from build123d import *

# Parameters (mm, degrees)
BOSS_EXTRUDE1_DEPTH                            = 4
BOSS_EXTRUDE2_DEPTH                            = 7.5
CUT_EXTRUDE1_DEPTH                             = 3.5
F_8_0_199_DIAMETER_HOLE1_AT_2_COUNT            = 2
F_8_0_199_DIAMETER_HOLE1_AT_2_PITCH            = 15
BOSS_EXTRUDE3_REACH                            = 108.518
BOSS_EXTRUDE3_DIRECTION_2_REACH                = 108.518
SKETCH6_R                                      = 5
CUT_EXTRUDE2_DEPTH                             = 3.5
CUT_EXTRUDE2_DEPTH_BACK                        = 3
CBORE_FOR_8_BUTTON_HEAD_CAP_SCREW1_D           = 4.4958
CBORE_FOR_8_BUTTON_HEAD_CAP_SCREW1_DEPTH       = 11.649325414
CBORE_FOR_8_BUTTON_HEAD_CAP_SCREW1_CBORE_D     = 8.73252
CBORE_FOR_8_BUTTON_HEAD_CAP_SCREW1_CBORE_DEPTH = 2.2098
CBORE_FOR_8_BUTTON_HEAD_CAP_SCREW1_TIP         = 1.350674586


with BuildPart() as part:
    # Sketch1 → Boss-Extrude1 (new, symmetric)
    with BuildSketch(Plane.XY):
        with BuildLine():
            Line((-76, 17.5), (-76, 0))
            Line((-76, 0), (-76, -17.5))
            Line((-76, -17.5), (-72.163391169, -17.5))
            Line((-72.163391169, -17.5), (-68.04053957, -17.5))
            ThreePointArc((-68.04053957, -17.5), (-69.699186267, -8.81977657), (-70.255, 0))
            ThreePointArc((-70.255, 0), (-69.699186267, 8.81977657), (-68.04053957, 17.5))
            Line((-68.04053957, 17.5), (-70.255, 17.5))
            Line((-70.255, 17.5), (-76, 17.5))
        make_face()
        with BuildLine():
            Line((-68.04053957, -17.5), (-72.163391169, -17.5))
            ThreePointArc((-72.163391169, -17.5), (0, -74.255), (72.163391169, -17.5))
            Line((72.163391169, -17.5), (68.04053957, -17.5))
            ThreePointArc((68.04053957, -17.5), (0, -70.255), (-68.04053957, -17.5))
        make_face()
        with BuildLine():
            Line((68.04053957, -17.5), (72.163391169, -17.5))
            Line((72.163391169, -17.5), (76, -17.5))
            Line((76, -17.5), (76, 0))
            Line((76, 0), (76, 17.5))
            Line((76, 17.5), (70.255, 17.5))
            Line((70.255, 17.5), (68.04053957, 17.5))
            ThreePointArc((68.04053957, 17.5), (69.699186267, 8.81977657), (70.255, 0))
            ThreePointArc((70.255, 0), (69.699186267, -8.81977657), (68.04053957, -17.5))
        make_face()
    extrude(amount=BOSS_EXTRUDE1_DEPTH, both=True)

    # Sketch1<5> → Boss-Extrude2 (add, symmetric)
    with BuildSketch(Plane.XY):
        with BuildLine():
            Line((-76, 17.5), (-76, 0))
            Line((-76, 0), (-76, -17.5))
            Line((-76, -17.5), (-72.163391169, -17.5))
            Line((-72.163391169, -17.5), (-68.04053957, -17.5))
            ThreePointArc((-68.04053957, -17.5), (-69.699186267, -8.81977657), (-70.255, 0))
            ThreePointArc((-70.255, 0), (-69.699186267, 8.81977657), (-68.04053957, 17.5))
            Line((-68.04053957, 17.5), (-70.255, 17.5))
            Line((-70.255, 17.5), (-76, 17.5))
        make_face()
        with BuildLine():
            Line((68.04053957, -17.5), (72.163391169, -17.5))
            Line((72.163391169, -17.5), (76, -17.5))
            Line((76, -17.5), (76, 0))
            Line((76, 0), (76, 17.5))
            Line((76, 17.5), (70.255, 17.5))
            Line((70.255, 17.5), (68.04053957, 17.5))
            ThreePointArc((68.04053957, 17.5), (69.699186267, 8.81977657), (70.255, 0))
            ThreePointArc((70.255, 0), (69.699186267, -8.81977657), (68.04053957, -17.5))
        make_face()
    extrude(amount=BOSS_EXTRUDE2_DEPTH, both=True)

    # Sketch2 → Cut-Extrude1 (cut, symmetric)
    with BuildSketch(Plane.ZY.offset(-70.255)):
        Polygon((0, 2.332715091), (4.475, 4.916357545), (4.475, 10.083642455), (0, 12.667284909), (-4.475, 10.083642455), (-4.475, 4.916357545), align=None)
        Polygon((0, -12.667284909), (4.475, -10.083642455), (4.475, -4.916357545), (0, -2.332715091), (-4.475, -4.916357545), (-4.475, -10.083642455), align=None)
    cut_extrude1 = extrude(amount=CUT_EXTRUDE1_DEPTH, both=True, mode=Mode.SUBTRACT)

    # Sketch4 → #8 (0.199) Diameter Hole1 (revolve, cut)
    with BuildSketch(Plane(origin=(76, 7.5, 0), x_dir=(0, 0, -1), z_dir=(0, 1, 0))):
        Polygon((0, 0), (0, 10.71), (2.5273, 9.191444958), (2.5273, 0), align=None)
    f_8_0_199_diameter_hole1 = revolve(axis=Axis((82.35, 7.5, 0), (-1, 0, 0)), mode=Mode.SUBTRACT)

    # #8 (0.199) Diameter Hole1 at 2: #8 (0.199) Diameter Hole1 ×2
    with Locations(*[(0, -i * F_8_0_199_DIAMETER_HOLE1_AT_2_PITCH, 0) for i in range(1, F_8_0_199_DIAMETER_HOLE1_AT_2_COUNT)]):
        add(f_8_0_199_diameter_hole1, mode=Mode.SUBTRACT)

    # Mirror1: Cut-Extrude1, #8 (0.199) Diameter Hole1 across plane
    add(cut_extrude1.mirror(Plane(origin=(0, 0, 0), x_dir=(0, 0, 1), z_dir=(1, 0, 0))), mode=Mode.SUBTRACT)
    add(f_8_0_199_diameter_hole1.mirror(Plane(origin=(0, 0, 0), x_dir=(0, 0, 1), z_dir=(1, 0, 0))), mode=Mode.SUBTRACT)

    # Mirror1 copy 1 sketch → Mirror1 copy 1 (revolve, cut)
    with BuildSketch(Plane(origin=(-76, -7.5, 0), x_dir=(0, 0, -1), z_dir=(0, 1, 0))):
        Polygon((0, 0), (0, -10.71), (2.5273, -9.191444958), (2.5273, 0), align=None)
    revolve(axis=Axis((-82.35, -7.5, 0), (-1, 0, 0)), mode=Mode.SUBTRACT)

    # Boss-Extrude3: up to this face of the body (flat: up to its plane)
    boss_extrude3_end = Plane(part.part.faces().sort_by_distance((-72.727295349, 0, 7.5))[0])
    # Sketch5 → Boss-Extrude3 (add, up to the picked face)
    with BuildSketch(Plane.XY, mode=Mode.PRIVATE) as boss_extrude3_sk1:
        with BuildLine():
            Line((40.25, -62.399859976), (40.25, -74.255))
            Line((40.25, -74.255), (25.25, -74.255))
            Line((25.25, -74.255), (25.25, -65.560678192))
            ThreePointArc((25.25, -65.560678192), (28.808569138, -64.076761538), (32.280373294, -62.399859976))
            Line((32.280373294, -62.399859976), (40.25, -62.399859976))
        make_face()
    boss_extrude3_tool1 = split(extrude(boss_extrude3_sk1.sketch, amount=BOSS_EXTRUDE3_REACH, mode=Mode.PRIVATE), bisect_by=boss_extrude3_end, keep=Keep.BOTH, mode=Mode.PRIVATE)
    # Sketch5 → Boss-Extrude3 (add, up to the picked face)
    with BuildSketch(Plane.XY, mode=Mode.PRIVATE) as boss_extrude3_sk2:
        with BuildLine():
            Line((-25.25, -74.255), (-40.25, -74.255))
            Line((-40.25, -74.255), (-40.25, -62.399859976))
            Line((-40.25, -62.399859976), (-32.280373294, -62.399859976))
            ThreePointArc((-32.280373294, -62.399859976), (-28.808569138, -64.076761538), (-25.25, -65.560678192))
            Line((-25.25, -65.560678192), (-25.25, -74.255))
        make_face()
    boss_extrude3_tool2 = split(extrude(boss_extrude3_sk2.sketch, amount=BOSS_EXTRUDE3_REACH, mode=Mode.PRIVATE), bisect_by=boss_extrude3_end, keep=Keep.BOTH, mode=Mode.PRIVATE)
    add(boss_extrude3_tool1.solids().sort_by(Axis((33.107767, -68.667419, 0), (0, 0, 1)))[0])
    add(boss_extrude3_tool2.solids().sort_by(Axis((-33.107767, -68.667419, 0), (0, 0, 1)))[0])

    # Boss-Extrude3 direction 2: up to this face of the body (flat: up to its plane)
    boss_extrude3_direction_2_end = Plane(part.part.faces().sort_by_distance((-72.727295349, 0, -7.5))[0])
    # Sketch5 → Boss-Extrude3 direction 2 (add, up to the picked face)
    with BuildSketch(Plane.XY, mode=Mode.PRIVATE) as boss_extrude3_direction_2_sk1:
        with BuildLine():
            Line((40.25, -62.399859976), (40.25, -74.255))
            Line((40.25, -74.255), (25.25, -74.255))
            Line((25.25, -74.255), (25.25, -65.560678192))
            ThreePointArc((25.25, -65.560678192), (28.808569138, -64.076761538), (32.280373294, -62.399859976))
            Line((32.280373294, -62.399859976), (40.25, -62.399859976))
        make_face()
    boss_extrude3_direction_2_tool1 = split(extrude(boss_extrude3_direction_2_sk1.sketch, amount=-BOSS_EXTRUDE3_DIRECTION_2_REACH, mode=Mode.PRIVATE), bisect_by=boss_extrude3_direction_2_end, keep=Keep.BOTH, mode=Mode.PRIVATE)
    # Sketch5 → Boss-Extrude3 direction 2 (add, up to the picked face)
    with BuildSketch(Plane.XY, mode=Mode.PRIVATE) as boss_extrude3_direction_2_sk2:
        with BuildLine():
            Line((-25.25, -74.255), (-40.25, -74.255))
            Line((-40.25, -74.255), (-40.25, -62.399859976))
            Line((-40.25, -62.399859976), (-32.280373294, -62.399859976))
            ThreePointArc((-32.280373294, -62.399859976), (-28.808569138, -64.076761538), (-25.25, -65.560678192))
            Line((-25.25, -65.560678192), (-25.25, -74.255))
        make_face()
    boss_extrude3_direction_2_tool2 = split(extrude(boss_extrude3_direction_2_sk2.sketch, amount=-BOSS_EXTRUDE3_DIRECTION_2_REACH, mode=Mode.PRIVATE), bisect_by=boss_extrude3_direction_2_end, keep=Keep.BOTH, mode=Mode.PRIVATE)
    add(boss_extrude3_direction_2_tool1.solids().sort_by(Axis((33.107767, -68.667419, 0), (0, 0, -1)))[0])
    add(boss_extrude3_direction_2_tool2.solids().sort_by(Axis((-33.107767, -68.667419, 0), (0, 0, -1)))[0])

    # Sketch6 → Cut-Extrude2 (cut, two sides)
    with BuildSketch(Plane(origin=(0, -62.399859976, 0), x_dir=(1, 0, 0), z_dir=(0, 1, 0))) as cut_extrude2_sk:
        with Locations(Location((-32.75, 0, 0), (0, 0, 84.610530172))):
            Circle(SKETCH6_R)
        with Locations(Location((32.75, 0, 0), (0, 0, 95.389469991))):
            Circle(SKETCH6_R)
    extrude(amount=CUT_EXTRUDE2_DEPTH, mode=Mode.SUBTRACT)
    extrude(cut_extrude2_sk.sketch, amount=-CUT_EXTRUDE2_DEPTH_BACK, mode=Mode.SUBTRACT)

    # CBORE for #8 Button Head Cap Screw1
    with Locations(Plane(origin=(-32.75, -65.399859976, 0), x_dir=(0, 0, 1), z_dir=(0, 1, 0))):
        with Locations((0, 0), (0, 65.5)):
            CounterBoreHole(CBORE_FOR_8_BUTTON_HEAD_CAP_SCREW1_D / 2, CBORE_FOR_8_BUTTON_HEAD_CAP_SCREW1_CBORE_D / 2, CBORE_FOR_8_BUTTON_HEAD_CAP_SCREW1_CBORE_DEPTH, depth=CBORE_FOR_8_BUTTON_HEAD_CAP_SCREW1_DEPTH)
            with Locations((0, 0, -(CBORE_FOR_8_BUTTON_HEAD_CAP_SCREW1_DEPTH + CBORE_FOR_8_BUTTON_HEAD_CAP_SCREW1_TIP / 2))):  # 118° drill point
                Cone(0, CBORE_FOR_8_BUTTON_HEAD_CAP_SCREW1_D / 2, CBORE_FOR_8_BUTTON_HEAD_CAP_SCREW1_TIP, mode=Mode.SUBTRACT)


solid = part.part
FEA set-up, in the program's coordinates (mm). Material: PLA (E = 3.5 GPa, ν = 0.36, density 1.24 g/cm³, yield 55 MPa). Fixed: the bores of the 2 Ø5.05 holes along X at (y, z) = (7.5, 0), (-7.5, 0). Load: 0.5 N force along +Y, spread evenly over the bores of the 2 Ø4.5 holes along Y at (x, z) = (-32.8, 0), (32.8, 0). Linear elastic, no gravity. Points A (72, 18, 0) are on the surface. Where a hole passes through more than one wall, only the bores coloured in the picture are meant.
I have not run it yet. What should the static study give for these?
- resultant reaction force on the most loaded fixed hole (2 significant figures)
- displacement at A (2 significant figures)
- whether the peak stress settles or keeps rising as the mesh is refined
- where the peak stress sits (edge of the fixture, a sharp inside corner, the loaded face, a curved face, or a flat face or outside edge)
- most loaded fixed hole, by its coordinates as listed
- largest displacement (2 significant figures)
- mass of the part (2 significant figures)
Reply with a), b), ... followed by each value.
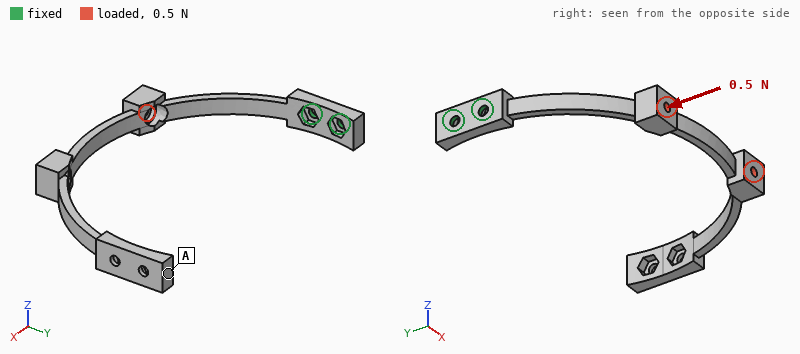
a) 3.4 N
b) 2.0 mm
c) keeps rising
d) a sharp inside corner
e) (7.5, 0)
f) 2.1 mm
g) 18 g
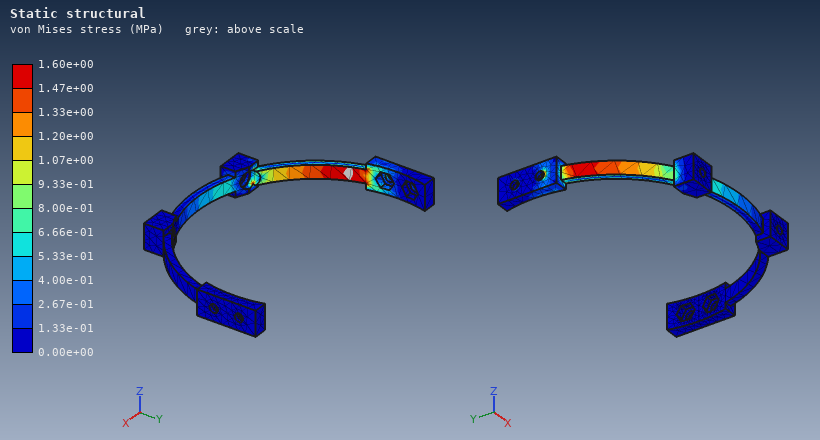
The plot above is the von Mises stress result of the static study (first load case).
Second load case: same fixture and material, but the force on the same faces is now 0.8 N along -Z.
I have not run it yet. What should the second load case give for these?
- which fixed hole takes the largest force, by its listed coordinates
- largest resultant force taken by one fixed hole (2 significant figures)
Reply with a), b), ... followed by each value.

a) (-7.5, 0)
b) 2.1 N
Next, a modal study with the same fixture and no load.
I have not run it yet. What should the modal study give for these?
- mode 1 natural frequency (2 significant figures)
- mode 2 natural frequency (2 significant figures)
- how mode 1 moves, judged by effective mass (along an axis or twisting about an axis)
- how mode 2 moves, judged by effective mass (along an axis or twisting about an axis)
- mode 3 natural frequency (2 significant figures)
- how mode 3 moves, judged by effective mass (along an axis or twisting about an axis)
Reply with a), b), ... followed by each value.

a) 19 Hz
b) 23 Hz
c) along Y
d) along Z
e) 58 Hz
f) along X
